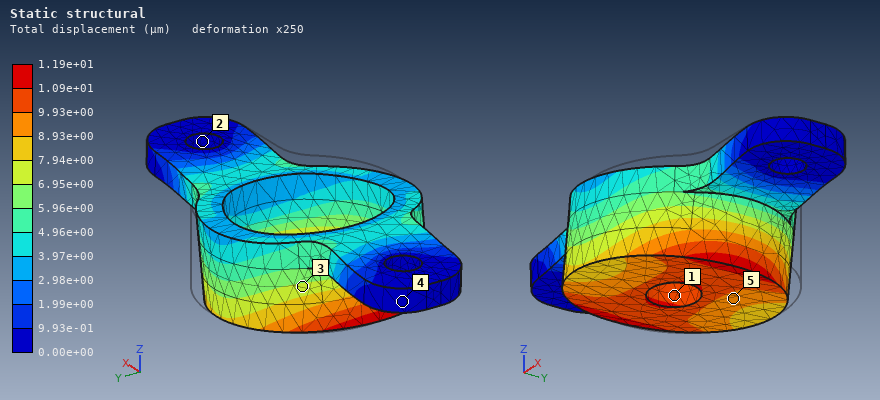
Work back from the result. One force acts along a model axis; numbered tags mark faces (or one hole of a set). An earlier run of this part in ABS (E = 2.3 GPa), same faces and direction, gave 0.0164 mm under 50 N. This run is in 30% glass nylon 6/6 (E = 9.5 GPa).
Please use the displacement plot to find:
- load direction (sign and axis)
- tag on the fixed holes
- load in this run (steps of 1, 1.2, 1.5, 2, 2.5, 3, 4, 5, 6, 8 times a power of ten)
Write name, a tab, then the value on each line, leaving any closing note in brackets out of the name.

load direction	-X
tag on the fixed holes	2
load in this run	150 N
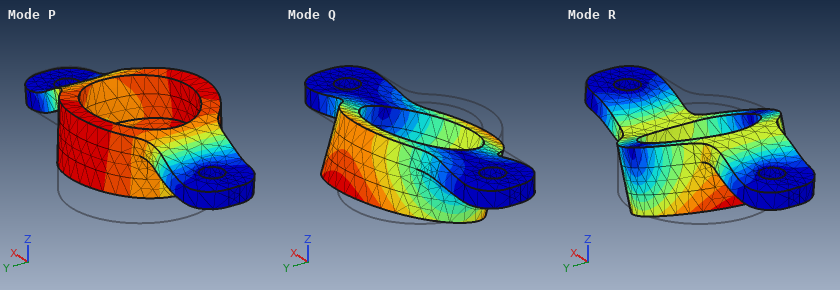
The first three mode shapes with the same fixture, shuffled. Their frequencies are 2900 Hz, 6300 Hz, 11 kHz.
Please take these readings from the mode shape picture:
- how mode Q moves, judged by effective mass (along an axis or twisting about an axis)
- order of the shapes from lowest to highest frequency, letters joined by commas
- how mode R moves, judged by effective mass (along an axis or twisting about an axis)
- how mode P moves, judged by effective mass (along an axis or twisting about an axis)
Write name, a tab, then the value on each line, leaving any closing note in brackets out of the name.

how mode Q moves, judged by effective mass	along Y
order of the shapes from lowest to highest frequency, letters joined by commas	Q, P, R
how mode R moves, judged by effective mass	along X
how mode P moves, judged by effective mass	along Z
